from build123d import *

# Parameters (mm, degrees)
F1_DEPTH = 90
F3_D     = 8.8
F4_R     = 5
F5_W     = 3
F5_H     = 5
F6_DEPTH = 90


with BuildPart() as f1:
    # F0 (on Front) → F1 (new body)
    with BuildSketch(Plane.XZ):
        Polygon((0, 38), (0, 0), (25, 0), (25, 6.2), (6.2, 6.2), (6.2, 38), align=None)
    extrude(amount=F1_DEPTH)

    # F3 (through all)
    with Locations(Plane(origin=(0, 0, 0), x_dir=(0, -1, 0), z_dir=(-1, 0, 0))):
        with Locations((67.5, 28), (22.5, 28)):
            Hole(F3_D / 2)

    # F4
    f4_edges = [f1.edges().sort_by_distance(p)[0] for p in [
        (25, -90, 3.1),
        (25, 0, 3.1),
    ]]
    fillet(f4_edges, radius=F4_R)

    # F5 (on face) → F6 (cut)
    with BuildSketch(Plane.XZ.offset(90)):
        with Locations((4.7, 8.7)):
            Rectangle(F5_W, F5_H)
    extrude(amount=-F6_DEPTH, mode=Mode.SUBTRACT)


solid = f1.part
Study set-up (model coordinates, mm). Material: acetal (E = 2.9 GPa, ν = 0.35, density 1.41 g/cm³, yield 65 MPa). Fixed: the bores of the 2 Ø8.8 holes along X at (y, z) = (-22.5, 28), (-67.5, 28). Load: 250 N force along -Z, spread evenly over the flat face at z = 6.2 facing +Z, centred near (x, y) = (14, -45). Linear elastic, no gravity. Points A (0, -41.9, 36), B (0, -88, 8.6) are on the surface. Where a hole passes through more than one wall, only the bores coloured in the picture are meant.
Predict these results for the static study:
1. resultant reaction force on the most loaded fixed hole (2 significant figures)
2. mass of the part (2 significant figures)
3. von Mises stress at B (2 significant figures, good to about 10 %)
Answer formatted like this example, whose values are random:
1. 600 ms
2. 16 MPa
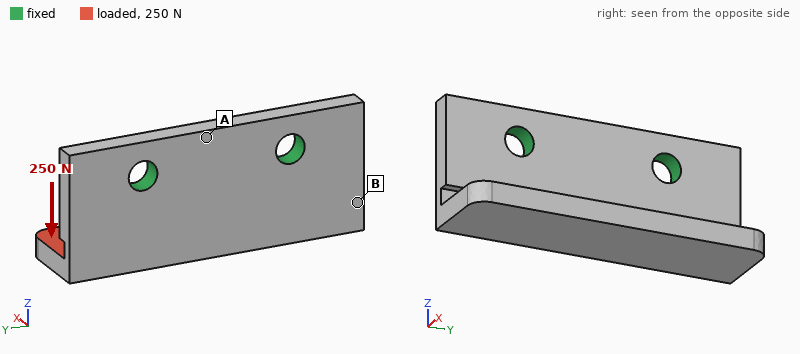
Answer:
1. 130 N
2. 42 g
3. 17 MPa
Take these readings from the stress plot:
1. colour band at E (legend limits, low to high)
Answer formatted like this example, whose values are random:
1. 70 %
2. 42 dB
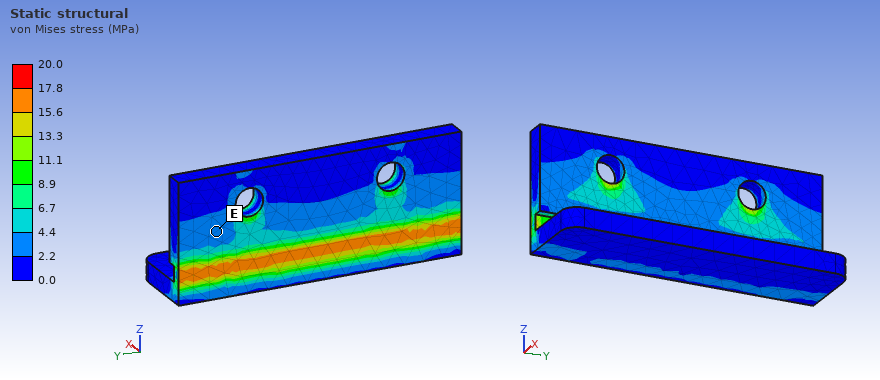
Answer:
1. 2.2 to 4.4 MPa
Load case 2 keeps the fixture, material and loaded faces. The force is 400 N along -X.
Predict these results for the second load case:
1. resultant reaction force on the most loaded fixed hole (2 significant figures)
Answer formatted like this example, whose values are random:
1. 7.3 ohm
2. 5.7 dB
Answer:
1. 200 N
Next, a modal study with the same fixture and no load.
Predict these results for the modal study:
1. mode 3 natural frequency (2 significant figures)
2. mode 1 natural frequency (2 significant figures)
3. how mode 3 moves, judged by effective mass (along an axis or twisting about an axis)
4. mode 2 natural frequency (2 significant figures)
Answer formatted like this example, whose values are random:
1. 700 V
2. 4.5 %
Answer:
1. 1700 Hz
2. 640 Hz
3. along X
4. 1100 Hz
